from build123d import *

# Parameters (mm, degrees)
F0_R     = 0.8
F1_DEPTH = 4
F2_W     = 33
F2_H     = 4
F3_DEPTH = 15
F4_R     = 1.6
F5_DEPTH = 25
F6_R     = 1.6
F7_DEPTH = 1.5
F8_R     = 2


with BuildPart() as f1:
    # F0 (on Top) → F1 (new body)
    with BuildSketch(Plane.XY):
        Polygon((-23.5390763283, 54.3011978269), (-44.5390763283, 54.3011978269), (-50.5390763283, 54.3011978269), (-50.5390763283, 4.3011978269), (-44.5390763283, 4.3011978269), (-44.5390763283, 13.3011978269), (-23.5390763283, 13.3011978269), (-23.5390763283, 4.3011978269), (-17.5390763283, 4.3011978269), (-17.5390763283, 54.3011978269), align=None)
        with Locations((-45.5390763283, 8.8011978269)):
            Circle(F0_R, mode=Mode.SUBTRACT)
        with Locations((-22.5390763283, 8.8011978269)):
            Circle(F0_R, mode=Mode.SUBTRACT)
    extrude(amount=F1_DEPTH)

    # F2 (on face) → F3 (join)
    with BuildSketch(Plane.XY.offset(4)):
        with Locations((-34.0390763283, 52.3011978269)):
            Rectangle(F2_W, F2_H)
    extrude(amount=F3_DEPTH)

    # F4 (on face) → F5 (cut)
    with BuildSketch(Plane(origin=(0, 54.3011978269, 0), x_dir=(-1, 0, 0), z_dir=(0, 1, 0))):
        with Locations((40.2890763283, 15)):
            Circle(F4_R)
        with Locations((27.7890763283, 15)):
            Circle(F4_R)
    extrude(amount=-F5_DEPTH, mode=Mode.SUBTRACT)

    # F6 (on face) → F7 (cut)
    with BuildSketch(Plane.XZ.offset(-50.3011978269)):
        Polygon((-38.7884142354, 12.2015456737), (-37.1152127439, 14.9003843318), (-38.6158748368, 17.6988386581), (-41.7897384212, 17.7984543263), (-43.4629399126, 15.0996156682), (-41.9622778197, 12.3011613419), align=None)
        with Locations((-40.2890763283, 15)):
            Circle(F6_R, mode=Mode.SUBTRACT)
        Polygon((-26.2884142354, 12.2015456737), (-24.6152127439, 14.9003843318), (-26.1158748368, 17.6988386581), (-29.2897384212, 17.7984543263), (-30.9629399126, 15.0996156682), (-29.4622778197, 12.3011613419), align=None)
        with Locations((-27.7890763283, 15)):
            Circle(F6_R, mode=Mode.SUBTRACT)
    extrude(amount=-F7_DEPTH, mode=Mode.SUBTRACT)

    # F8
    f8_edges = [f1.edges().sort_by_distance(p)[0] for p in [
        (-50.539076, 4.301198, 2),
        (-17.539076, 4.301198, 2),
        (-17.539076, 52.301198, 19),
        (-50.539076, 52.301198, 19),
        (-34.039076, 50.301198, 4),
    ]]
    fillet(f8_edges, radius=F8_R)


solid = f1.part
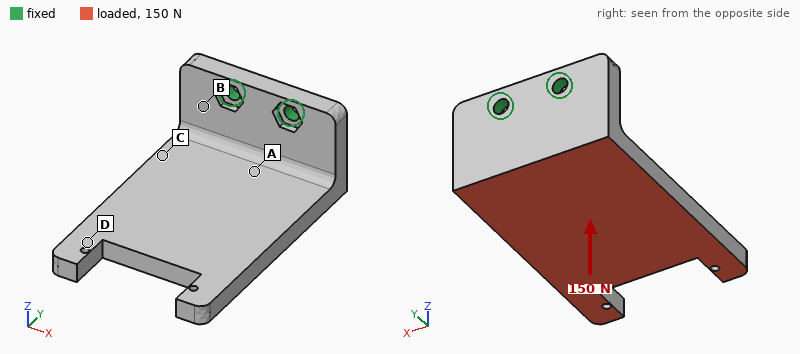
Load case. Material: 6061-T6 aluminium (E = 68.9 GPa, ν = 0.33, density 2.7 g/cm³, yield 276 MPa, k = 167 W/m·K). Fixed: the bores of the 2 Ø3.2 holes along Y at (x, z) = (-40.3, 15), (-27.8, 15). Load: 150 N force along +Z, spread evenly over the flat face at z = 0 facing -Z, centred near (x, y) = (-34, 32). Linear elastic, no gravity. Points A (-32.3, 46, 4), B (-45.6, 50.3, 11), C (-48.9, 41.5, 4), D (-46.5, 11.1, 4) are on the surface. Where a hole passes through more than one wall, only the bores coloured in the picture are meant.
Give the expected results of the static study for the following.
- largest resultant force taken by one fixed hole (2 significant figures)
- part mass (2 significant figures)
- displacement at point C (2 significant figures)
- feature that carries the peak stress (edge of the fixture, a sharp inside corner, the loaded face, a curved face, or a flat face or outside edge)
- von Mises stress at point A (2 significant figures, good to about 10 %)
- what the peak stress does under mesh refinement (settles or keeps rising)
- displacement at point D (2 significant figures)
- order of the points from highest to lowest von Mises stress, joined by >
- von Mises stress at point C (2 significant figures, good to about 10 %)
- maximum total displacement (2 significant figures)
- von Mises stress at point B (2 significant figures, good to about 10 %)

75 N
21 g
0.059 mm
edge of the fixture
23 MPa
keeps rising
0.26 mm
B > A > C > D
19 MPa
0.31 mm
35 MPa
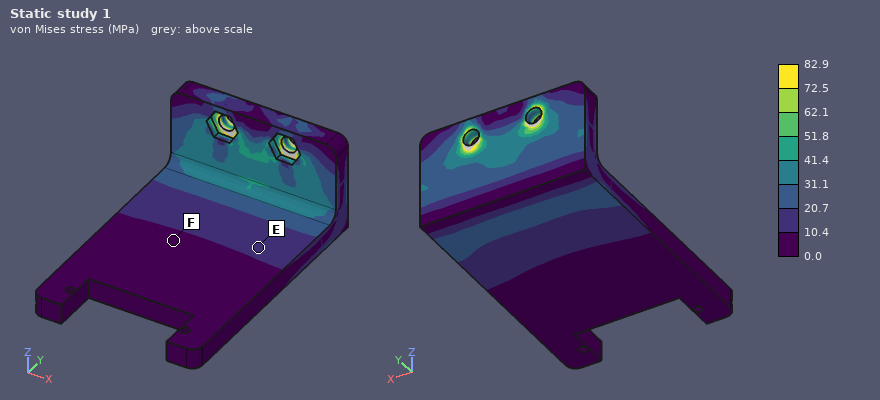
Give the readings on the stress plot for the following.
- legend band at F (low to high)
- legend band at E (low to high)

0.0 to 10.4 MPa
10.4 to 20.7 MPa
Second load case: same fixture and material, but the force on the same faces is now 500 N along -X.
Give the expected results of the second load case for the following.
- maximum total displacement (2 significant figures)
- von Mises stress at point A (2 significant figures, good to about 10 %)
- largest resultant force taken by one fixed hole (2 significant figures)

0.23 mm
27 MPa
880 N
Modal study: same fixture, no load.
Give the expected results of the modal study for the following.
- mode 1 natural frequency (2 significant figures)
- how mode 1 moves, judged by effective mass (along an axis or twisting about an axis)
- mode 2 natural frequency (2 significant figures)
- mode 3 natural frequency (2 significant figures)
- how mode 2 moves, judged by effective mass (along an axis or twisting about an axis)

1100 Hz
along Z
2200 Hz
4400 Hz
along X
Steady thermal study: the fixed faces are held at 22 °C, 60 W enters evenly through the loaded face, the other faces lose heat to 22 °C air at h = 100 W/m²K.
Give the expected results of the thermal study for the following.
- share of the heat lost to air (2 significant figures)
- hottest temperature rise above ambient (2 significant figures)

23 %
71 K
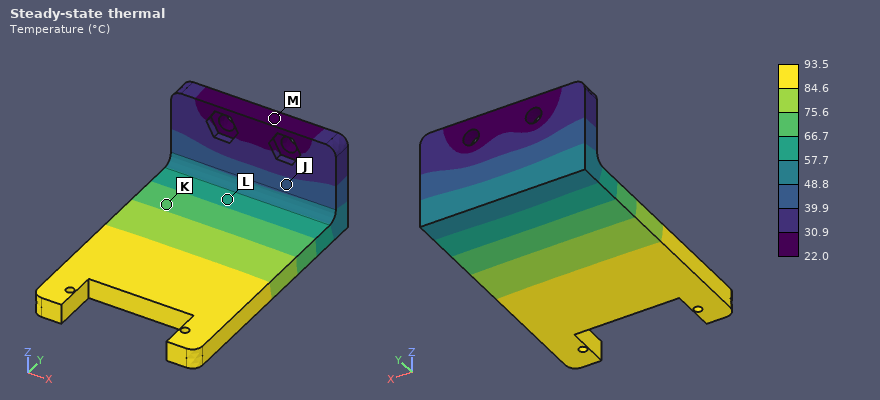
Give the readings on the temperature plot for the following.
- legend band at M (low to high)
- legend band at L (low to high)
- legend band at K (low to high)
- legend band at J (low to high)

22.0 to 30.9 °C
57.7 to 66.7 °C
66.7 to 75.6 °C
39.9 to 48.8 °C
